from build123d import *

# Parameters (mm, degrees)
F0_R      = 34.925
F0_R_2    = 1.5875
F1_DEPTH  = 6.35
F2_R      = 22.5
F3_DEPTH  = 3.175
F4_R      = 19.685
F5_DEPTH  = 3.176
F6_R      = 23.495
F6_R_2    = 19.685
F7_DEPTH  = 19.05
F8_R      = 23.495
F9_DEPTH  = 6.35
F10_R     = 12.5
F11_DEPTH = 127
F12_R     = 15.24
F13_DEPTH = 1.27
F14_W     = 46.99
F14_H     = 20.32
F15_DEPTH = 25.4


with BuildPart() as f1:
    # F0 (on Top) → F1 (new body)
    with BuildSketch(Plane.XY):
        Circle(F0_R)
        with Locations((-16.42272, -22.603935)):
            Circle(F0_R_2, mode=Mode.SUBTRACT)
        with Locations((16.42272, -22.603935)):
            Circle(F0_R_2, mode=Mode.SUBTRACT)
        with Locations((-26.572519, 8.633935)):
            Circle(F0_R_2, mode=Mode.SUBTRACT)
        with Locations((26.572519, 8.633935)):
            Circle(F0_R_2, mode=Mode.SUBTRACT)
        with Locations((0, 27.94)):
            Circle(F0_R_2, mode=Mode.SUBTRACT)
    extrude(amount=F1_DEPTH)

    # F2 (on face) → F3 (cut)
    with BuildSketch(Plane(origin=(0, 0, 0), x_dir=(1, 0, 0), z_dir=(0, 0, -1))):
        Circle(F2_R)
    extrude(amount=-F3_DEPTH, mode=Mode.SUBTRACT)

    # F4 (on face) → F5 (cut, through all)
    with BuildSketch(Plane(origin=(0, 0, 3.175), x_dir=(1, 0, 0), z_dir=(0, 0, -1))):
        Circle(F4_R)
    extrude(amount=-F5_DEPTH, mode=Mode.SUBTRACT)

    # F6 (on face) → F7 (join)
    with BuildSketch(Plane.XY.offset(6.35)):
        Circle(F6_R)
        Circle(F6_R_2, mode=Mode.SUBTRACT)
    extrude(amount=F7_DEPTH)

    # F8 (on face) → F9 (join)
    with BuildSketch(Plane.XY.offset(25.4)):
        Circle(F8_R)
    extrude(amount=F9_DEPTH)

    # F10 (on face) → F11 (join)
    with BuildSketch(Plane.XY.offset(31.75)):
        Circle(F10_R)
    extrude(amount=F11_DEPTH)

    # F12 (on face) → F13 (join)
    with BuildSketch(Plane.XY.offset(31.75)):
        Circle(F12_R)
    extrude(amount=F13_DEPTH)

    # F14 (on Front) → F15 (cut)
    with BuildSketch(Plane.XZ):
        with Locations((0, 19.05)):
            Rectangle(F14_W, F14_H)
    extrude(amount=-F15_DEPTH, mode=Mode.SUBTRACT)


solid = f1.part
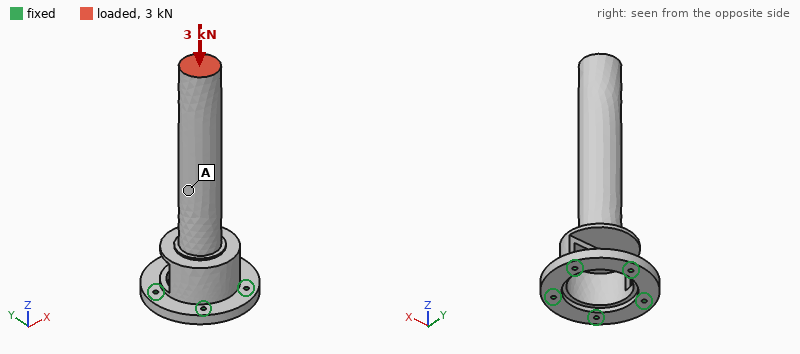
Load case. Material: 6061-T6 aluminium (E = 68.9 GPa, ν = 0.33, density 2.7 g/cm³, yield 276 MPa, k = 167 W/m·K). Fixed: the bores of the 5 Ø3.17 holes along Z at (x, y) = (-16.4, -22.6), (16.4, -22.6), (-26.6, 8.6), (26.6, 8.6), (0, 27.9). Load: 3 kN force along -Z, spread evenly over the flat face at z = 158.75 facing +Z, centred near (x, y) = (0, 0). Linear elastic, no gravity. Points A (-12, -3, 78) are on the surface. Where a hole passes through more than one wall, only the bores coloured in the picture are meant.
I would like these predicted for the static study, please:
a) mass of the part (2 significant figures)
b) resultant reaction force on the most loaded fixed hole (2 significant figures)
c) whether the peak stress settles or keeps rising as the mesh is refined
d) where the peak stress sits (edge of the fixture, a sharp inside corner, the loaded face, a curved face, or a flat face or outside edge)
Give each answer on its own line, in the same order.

250 g
1.2 kN
keeps rising
edge of the fixture
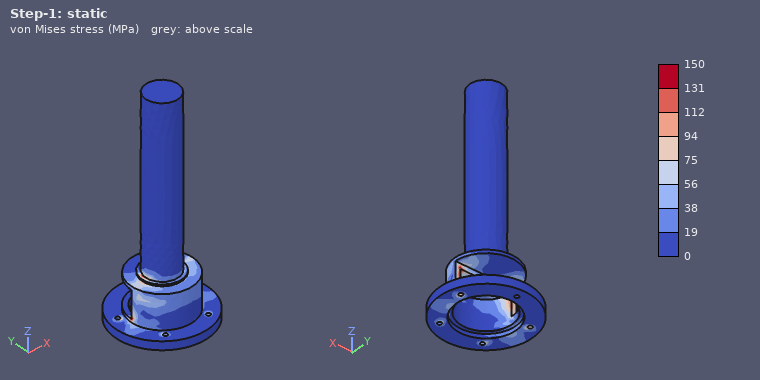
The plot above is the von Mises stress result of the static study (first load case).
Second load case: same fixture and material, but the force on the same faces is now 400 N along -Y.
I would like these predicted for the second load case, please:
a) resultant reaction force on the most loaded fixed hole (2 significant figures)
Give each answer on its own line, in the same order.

1.2 kN
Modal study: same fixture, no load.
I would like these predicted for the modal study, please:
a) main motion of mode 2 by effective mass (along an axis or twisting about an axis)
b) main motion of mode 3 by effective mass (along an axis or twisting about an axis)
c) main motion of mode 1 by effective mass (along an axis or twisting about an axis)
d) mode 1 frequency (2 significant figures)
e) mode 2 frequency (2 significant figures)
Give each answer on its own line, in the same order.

along X
along X
along Y
370 Hz
640 Hz
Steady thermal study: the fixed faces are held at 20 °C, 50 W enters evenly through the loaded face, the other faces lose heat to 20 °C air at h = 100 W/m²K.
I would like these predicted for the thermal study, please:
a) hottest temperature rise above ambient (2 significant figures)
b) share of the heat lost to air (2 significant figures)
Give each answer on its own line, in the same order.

59 K
75 %
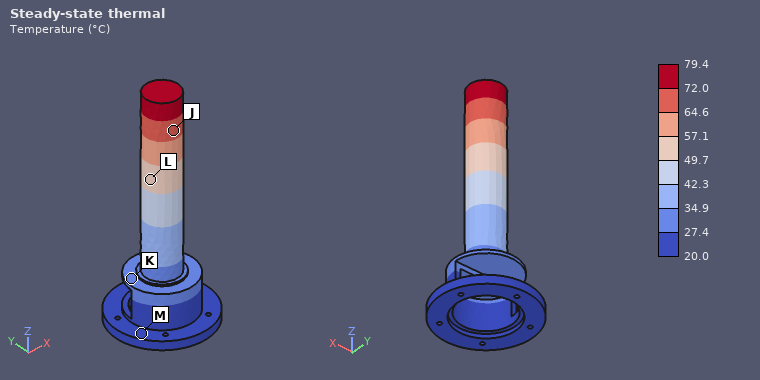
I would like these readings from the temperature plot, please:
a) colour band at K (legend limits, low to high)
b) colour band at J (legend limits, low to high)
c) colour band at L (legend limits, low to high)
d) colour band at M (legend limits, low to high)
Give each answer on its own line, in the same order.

27.4 to 34.9 °C
64.6 to 72.0 °C
49.7 to 57.1 °C
20.0 to 27.4 °C
